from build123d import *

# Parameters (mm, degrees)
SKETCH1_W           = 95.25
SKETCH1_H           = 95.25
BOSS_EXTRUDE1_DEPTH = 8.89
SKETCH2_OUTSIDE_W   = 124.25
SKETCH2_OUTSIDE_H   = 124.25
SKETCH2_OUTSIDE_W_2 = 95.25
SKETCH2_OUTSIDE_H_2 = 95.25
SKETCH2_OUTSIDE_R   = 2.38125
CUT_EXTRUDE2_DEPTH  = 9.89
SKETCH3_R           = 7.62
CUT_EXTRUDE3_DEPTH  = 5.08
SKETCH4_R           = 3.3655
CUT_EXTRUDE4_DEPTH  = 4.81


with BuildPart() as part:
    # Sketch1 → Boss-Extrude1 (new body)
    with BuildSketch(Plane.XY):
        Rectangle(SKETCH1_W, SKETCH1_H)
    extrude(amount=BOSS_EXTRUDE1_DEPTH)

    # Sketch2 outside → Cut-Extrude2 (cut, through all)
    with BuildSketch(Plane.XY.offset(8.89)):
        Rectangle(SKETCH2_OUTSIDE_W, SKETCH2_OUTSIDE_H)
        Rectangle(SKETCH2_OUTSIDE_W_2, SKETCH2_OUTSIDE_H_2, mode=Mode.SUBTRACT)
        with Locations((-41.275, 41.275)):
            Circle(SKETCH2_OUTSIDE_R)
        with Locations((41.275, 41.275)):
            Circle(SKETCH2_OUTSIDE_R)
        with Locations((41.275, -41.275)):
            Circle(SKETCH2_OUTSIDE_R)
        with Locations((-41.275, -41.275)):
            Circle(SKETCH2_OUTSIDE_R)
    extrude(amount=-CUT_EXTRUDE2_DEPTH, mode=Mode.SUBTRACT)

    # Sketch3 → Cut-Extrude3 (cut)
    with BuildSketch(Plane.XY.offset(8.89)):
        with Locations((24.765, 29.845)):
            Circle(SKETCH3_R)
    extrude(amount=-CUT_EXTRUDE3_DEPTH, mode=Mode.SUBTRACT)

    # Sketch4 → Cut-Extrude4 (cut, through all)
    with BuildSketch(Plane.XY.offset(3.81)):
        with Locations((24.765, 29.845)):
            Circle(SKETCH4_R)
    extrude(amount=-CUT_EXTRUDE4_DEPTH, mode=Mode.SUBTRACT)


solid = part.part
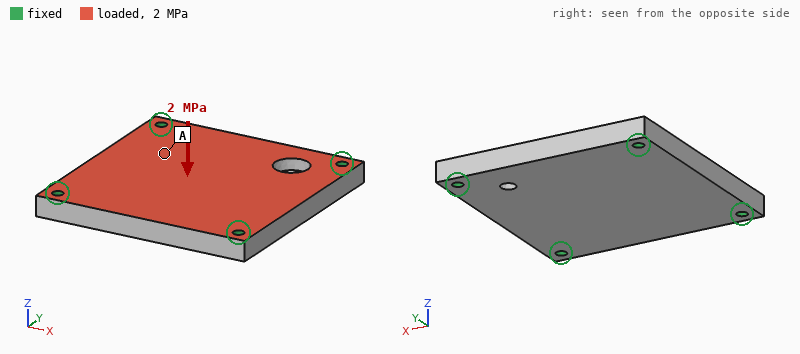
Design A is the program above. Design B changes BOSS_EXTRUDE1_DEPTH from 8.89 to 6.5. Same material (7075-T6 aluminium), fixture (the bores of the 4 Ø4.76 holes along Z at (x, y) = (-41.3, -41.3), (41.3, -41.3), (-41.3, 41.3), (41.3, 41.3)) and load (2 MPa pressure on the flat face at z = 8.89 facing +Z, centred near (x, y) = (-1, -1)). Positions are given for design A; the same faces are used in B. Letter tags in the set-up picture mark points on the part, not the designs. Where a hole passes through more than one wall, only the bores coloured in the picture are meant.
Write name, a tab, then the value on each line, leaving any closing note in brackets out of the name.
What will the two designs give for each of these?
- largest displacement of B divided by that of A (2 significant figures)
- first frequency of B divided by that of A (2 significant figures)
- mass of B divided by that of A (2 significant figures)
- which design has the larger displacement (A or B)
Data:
largest displacement of B divided by that of A	2.3
first frequency of B divided by that of A	0.77
mass of B divided by that of A	0.73
which design has the larger displacement	B
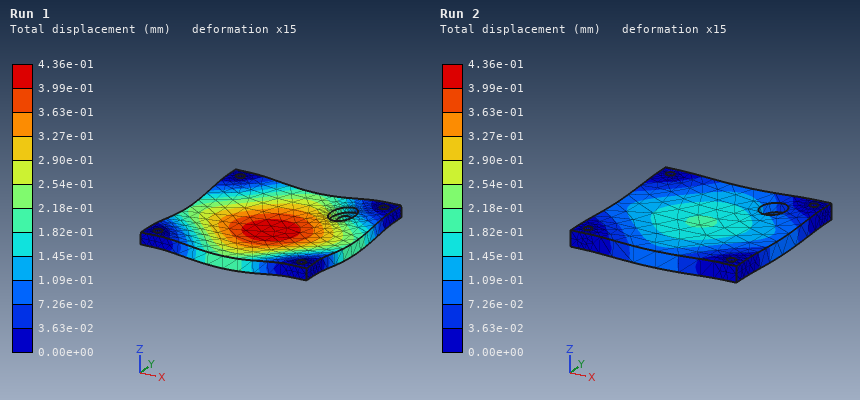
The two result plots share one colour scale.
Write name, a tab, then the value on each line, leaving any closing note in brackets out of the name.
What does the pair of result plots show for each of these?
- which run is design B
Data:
which run is design B	Run 1
